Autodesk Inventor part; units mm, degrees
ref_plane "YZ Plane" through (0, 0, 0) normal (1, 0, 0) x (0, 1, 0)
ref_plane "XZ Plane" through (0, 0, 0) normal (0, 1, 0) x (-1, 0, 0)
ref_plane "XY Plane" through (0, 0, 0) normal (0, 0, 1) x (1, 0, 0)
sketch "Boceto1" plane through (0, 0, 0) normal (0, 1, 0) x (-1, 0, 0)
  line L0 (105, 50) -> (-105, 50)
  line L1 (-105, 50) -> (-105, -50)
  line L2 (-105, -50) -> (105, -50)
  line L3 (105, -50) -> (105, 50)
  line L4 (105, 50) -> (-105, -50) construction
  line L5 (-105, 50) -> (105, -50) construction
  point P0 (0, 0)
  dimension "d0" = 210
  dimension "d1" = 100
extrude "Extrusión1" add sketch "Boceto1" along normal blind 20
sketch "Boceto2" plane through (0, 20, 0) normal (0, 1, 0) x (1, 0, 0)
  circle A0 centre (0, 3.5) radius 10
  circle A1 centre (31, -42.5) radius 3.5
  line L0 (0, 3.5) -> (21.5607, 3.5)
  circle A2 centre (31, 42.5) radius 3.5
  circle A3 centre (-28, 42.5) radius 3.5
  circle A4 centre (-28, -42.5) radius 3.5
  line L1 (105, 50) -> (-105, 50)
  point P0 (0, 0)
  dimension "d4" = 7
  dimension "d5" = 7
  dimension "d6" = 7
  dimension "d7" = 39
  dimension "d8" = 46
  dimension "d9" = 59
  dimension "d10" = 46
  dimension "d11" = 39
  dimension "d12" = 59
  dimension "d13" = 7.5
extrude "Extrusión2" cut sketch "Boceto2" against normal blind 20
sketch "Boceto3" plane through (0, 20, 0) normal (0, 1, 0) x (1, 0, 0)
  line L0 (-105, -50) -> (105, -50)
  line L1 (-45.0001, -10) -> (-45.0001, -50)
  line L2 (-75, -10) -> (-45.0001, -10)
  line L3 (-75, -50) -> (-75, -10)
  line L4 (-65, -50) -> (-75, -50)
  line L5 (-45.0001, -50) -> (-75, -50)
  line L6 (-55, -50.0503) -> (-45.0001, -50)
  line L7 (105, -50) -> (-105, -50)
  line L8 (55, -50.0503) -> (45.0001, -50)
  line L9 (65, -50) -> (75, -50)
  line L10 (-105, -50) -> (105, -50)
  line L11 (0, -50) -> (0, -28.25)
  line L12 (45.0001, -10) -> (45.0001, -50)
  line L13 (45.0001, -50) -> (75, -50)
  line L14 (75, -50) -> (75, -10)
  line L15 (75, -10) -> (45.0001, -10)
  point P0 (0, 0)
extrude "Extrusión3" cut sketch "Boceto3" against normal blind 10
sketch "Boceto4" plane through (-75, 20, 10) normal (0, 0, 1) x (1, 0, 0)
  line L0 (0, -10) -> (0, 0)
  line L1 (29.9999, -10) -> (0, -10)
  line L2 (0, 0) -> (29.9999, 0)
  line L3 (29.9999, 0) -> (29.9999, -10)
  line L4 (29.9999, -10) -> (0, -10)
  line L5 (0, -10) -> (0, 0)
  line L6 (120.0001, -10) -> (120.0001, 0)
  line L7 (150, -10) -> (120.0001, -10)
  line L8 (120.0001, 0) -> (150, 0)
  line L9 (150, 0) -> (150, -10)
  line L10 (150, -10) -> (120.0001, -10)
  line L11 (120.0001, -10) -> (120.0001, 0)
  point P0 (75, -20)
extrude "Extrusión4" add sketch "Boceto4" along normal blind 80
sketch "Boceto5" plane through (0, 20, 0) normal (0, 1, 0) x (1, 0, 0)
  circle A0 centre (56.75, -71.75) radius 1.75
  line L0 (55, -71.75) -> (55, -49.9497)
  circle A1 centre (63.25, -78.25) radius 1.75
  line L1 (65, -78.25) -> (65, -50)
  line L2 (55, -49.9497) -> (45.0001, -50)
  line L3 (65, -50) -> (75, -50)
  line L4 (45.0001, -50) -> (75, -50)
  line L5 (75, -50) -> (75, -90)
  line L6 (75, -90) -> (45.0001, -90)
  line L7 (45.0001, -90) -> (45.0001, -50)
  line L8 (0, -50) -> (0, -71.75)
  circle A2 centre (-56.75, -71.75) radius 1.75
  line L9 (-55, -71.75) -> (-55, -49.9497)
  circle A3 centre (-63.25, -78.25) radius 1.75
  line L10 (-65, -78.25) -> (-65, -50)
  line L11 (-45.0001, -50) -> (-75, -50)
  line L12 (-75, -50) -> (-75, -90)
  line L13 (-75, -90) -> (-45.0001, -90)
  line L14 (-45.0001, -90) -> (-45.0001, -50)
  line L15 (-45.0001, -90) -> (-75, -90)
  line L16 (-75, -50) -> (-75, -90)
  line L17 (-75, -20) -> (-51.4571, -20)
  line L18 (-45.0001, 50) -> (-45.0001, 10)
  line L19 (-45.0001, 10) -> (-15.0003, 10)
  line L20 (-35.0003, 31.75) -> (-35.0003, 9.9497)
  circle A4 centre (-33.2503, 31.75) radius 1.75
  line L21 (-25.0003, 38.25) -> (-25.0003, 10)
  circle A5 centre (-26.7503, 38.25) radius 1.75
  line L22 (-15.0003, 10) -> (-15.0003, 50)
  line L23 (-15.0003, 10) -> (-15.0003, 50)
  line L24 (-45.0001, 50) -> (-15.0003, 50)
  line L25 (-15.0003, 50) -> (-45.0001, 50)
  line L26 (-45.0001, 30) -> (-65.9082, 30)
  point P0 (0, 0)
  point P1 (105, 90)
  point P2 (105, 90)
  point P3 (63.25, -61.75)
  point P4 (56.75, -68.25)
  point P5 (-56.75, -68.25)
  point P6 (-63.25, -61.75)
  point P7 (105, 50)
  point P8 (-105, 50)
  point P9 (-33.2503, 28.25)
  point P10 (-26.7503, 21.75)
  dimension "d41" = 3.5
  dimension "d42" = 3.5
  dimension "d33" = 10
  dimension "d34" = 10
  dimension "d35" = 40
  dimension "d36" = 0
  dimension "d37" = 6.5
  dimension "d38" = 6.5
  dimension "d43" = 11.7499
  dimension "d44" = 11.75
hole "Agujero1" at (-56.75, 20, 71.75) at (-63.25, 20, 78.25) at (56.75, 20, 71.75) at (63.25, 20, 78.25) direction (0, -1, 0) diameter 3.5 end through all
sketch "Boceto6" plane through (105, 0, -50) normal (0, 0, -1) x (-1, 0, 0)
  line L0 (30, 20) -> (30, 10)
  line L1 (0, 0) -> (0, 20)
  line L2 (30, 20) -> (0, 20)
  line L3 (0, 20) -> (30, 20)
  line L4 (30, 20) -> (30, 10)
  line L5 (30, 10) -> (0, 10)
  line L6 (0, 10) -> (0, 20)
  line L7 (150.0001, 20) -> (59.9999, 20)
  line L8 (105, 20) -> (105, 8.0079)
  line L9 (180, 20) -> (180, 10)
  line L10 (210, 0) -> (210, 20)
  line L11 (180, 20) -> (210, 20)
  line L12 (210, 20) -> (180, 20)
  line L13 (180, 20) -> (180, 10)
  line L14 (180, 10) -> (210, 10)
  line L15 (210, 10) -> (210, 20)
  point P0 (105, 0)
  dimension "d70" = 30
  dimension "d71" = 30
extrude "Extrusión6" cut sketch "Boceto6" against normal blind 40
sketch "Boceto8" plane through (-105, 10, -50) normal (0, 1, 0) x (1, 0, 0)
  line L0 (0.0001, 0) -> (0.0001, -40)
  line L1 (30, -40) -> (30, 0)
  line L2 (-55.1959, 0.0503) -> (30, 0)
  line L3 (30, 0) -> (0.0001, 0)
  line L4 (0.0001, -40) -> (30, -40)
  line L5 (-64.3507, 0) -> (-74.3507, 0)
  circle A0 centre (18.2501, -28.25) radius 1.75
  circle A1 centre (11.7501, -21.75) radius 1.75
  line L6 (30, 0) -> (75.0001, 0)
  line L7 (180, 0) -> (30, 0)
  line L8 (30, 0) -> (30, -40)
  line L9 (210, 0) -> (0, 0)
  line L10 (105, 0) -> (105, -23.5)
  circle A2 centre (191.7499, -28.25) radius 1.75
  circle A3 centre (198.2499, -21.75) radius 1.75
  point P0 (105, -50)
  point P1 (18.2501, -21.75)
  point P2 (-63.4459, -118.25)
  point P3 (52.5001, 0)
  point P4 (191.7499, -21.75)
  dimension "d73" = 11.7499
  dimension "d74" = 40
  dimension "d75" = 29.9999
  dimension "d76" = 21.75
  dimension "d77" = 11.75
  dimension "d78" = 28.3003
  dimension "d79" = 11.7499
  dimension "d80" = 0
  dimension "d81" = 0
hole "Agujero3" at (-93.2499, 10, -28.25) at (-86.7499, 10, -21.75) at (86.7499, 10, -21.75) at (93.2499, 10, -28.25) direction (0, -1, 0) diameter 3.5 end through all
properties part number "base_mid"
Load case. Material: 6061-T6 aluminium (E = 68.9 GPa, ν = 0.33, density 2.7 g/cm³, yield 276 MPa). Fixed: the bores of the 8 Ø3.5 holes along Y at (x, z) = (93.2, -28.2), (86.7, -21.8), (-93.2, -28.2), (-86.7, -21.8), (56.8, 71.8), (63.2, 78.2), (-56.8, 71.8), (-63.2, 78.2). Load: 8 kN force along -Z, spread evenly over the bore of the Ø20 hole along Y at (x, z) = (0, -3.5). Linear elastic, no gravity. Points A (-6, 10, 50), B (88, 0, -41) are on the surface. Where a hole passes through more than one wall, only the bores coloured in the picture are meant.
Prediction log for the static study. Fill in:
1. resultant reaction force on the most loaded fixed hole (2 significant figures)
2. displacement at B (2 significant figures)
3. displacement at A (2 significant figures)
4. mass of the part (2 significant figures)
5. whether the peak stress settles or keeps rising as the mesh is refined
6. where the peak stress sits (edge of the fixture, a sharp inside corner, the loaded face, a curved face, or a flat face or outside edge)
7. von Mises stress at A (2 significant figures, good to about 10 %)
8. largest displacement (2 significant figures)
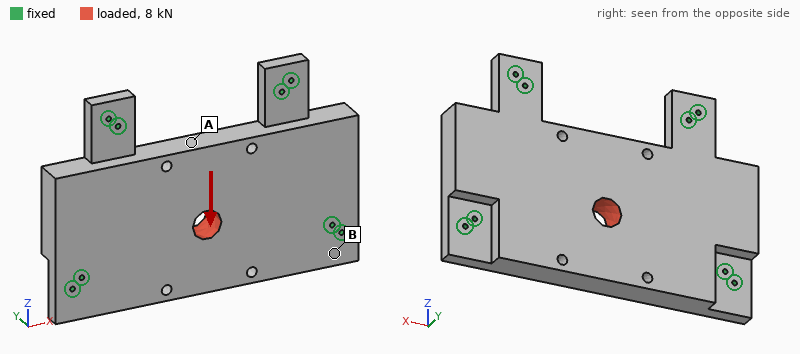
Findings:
1.5 kN
2.2 µm
11 µm
1.1 kg
keeps rising
edge of the fixture
7.0 MPa
14 µm
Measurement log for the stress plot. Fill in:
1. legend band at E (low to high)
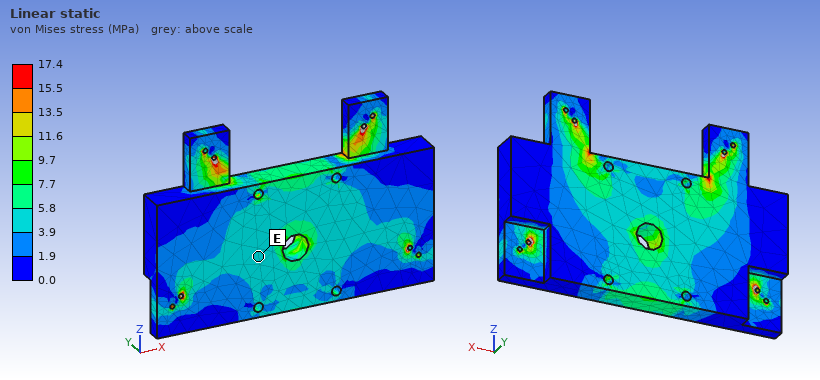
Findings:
3.9 to 5.8 MPa
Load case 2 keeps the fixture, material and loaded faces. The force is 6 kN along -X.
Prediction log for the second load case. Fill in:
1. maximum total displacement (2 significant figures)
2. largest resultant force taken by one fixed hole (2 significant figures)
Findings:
5.8 µm
1.6 kN
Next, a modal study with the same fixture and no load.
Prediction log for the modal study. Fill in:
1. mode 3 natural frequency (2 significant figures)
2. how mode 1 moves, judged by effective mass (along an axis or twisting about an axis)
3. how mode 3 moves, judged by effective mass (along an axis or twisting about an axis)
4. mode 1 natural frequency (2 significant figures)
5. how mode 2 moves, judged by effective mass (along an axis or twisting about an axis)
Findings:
3900 Hz
along Y
twisting about Z
2000 Hz
along Y
